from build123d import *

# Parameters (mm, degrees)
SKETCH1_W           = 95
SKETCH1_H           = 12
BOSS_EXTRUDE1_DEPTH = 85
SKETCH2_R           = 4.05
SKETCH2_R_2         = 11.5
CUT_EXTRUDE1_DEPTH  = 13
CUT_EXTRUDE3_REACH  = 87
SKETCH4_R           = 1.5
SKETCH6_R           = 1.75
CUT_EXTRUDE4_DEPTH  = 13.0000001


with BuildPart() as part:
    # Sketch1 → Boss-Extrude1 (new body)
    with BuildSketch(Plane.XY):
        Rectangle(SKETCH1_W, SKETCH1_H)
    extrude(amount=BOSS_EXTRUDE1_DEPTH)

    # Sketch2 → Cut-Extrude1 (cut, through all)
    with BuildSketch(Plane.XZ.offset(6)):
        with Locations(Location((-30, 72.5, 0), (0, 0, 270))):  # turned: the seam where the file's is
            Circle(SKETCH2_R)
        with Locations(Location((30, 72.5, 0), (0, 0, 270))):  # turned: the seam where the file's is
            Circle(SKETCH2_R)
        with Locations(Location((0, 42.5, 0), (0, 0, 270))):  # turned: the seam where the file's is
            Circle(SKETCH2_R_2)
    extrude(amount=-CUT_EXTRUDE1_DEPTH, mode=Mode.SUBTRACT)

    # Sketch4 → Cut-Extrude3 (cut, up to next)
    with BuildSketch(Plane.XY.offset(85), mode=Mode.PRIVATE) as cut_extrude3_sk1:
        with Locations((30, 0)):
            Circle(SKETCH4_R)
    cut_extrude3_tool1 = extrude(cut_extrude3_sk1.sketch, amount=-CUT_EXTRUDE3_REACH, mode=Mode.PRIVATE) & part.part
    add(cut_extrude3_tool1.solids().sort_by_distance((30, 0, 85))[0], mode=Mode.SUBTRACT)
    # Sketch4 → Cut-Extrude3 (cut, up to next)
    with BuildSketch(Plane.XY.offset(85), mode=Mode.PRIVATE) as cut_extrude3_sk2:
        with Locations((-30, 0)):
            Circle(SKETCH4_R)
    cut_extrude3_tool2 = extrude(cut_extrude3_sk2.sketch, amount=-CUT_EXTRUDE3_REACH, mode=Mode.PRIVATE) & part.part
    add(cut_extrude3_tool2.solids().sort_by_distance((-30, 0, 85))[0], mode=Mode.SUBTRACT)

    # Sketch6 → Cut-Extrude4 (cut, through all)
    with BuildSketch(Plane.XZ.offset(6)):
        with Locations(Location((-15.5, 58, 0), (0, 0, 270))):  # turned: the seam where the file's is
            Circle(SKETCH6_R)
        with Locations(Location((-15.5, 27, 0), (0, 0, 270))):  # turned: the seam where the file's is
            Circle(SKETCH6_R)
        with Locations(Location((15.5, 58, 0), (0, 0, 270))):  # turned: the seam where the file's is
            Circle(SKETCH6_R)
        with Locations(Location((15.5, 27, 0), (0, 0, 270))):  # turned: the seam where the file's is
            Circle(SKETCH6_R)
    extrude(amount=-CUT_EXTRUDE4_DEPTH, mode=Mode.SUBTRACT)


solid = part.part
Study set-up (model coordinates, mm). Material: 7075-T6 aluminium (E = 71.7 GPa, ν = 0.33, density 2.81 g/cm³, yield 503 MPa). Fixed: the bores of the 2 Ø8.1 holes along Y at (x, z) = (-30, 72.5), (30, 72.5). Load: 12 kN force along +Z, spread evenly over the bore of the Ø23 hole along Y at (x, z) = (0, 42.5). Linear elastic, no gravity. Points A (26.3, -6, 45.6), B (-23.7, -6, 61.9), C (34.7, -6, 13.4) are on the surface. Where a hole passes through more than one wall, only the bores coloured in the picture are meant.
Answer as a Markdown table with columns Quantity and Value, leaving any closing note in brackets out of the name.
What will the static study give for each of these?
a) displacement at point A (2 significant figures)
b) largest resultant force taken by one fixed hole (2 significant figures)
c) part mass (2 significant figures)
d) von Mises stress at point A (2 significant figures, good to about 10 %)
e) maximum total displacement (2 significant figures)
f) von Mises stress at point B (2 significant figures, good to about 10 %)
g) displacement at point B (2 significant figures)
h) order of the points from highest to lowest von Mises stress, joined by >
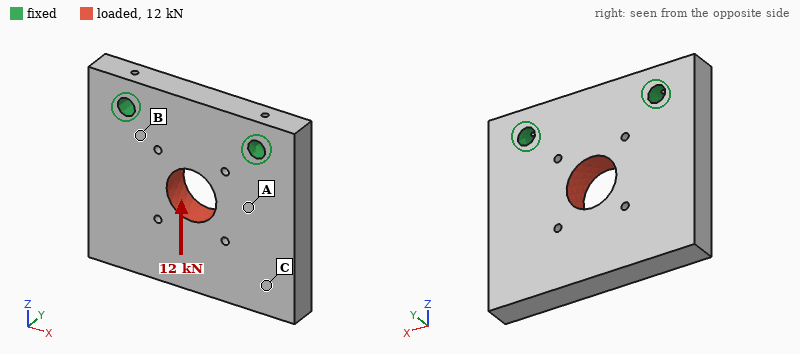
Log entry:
| Quantity | Value |
|---|---|
| displacement at point A | 5.7 µm |
| largest resultant force taken by one fixed hole | 6.2 kN |
| part mass | 250 g |
| von Mises stress at point A | 12 MPa |
| maximum total displacement | 14 µm |
| von Mises stress at point B | 23 MPa |
| displacement at point B | 3.5 µm |
| order of the points from highest to lowest von Mises stress, joined by > | B > A > C |
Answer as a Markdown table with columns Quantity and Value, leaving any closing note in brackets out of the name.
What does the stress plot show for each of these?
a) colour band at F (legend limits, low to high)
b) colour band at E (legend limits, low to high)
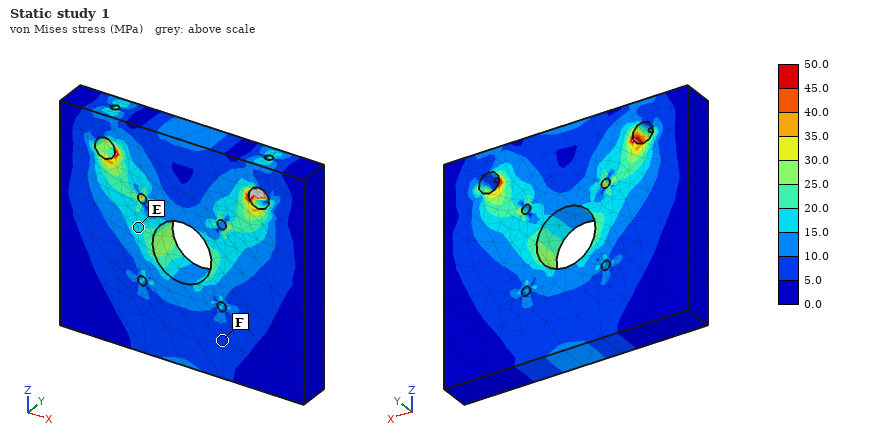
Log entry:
| Quantity | Value |
|---|---|
| colour band at F | 5.0 to 10.0 MPa |
| colour band at E | 15.0 to 20.0 MPa |
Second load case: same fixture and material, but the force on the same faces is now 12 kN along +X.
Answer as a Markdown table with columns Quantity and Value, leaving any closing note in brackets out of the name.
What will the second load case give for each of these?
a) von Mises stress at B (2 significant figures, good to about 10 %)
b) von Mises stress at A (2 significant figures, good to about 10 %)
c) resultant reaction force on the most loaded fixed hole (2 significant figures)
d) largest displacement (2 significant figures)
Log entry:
| Quantity | Value |
|---|---|
| von Mises stress at B | 27 MPa |
| von Mises stress at A | 19 MPa |
| resultant reaction force on the most loaded fixed hole | 8.0 kN |
| largest displacement | 36 µm |
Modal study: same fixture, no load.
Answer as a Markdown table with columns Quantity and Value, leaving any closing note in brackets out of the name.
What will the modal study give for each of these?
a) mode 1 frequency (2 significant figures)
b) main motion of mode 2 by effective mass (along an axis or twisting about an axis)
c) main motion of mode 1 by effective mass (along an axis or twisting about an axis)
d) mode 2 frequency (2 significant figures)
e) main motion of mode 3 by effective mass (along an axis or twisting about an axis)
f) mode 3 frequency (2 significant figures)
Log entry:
| Quantity | Value |
|---|---|
| mode 1 frequency | 1600 Hz |
| main motion of mode 2 by effective mass | twisting about Z |
| main motion of mode 1 by effective mass | along Y |
| mode 2 frequency | 3300 Hz |
| main motion of mode 3 by effective mass | along X |
| mode 3 frequency | 6300 Hz |
